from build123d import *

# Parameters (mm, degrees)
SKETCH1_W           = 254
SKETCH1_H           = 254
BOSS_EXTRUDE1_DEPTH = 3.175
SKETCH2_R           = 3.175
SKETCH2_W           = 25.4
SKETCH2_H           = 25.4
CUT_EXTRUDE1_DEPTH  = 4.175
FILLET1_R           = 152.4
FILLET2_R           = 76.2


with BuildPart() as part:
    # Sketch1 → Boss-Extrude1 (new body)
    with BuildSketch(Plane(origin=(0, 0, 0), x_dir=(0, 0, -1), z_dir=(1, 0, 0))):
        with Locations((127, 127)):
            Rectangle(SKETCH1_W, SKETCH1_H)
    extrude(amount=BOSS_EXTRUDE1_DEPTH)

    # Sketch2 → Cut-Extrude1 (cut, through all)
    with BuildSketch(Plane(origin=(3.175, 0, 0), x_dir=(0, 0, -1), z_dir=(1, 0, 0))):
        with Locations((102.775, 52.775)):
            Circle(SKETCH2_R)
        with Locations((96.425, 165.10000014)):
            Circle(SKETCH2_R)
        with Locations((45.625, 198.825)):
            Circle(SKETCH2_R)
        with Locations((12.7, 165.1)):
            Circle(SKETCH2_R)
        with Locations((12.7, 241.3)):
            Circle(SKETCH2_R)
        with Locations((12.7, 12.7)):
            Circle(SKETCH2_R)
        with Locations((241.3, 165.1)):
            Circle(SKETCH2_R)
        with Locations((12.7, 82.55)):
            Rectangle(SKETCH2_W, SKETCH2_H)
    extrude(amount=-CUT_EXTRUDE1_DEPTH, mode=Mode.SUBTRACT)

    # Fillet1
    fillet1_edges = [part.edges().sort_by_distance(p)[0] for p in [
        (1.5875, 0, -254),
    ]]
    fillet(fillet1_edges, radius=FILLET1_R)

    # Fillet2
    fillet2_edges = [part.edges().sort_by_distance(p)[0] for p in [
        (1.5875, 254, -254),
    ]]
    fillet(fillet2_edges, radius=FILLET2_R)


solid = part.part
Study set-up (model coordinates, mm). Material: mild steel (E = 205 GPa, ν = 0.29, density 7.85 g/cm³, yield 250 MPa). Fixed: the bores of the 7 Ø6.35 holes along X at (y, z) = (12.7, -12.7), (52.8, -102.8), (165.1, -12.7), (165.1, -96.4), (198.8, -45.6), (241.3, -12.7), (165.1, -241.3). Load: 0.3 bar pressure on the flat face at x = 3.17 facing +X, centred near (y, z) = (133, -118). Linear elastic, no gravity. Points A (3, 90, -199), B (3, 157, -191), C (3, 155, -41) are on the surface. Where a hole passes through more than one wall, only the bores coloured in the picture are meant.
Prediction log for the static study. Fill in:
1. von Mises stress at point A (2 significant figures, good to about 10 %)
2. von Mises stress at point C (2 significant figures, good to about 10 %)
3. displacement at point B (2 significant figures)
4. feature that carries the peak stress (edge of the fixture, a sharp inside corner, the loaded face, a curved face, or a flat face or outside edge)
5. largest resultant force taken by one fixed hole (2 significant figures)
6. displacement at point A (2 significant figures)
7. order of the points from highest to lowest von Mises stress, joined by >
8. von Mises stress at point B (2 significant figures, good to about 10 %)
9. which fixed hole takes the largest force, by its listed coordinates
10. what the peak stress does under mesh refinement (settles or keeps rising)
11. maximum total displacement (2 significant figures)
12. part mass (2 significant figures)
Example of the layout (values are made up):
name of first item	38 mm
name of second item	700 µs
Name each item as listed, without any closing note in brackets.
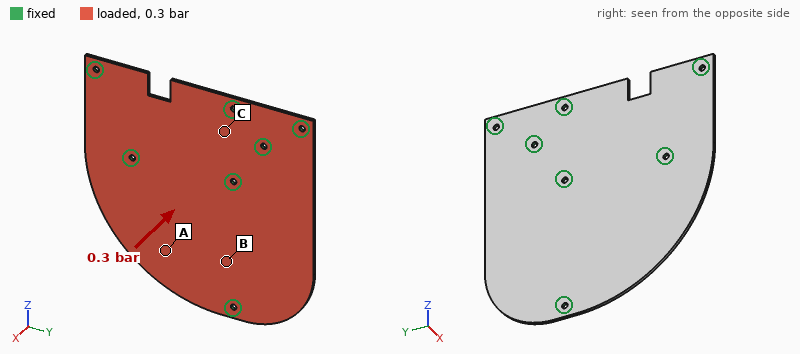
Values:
von Mises stress at point A	24 MPa
von Mises stress at point C	8.5 MPa
displacement at point B	0.10 mm
feature that carries the peak stress	edge of the fixture
largest resultant force taken by one fixed hole	470 N
displacement at point A	0.23 mm
order of the points from highest to lowest von Mises stress, joined by >	B > A > C
von Mises stress at point B	35 MPa
which fixed hole takes the largest force, by its listed coordinates	(52.8, -102.8)
what the peak stress does under mesh refinement	keeps rising
maximum total displacement	0.40 mm
part mass	1.4 kg
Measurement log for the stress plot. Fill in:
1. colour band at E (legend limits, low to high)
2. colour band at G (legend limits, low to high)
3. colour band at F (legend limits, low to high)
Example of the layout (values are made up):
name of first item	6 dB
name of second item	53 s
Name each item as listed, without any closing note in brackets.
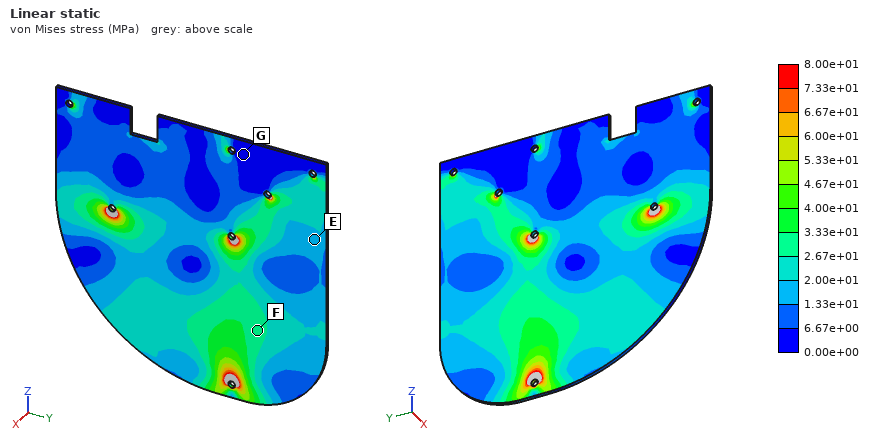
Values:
colour band at E	1.33e+01 to 2.00e+01 MPa
colour band at G	0.00e+00 to 6.67e+00 MPa
colour band at F	2.67e+01 to 3.33e+01 MPa
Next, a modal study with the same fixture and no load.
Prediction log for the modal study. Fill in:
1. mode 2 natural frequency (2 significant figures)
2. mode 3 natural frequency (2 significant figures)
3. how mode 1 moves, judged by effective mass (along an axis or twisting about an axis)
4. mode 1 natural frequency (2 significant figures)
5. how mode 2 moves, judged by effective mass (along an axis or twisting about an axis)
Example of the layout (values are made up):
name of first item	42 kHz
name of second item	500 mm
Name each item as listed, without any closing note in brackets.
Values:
mode 2 natural frequency	370 Hz
mode 3 natural frequency	730 Hz
how mode 1 moves, judged by effective mass	twisting about Z
mode 1 natural frequency	330 Hz
how mode 2 moves, judged by effective mass	along X
